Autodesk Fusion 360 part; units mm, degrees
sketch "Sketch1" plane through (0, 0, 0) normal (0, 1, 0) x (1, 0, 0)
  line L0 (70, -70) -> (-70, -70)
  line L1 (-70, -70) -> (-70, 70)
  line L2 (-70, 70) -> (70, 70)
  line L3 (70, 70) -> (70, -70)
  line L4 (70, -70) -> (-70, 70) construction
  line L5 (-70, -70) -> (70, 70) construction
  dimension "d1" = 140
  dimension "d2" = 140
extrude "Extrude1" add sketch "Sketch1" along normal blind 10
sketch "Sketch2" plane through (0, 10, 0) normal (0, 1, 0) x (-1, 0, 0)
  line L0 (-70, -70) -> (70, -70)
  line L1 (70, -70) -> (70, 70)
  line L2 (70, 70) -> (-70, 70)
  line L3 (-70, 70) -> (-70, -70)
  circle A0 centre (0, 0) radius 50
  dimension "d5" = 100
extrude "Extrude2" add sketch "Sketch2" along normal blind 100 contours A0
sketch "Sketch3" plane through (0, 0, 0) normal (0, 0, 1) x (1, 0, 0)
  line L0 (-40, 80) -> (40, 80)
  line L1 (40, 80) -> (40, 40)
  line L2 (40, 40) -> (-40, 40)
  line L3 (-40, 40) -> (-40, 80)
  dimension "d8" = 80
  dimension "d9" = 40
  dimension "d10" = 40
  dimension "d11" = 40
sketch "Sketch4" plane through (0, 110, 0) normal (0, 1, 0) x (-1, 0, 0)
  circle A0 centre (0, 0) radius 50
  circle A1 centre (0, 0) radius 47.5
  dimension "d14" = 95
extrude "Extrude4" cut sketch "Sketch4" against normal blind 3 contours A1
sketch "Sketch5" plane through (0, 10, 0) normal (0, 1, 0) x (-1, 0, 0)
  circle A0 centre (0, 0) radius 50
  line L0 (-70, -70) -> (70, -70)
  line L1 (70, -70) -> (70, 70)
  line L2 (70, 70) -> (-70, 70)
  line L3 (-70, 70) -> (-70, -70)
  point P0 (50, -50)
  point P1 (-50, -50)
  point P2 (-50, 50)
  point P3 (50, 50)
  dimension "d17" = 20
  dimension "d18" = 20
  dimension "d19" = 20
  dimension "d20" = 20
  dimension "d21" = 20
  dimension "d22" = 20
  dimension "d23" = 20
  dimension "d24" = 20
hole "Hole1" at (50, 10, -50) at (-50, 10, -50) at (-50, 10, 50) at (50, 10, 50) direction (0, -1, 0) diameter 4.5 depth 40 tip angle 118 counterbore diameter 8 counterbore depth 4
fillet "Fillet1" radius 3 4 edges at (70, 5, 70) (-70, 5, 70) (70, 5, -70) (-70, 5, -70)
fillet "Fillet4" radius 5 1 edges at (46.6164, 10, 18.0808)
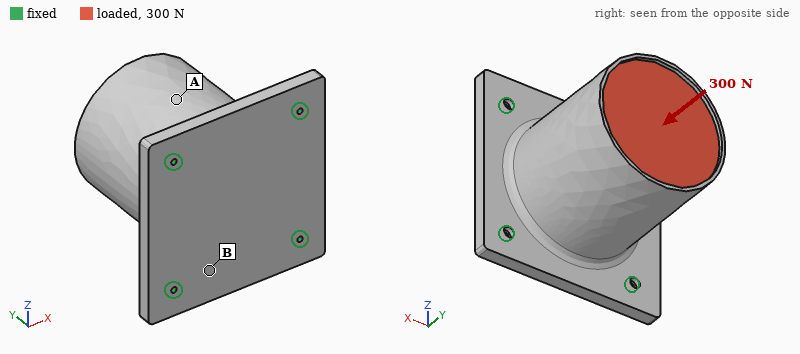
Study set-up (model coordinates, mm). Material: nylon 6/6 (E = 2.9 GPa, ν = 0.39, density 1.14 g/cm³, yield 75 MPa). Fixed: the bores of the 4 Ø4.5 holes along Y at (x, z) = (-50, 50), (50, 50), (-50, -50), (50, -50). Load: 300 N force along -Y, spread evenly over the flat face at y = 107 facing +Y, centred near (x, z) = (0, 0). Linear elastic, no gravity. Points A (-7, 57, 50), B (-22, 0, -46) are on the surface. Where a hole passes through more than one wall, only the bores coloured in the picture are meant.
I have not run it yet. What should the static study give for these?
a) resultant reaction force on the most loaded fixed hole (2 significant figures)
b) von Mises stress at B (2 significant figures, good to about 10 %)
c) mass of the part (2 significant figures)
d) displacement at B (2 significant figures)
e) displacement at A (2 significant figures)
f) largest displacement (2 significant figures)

98 N
0.48 MPa
1.1 kg
21 µm
23 µm
24 µm
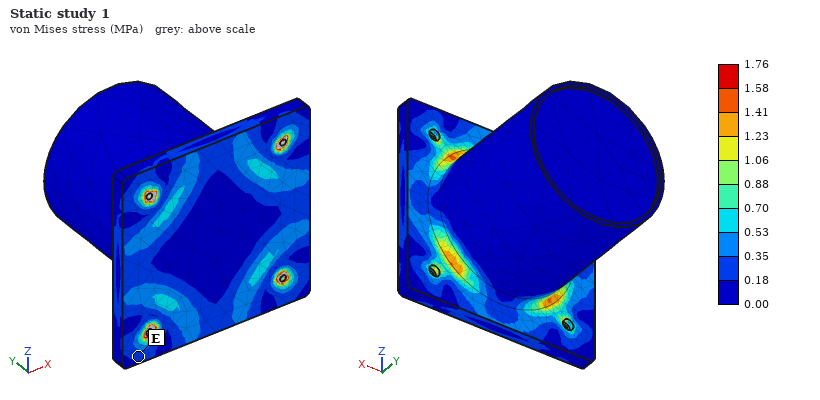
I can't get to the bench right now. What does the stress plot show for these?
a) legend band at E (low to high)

0.18 to 0.35 MPa
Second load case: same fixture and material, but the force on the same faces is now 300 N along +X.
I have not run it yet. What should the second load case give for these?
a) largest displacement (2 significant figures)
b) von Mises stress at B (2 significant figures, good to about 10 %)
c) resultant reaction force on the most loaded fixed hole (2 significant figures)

0.13 mm
1.1 MPa
200 N
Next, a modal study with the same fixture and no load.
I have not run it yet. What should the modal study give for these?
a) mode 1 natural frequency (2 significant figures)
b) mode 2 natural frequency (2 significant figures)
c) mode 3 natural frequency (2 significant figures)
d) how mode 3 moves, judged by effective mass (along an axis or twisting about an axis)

420 Hz
420 Hz
570 Hz
along Y
